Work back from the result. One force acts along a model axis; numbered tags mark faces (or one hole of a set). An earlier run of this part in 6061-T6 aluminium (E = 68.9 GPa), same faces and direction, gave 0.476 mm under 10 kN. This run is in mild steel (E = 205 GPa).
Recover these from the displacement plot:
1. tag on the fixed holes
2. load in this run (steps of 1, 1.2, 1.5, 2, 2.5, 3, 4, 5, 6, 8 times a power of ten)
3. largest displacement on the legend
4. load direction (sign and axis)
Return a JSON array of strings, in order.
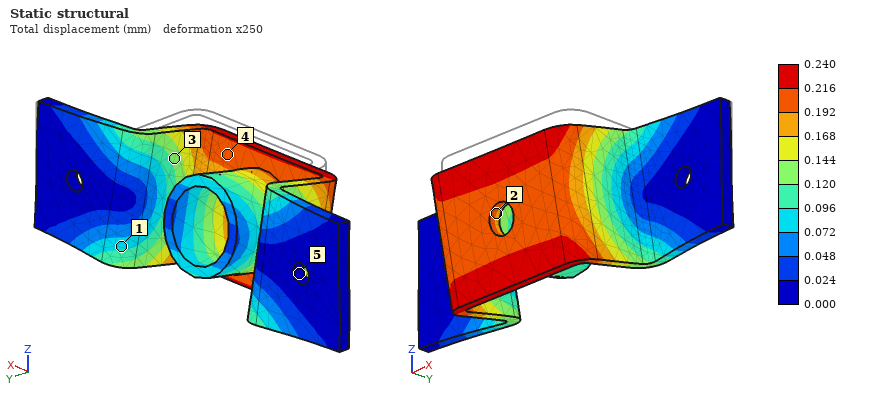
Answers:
["5", "15 kN", "0.240 mm", "-Z"]
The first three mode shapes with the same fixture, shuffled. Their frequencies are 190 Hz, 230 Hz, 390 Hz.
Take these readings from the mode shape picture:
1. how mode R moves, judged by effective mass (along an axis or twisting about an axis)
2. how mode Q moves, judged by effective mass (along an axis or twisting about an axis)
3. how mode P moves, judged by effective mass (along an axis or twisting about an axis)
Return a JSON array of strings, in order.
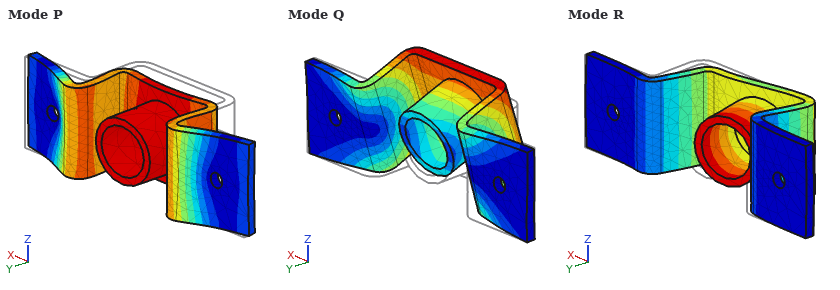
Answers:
["along X", "along Z", "along Y"]
